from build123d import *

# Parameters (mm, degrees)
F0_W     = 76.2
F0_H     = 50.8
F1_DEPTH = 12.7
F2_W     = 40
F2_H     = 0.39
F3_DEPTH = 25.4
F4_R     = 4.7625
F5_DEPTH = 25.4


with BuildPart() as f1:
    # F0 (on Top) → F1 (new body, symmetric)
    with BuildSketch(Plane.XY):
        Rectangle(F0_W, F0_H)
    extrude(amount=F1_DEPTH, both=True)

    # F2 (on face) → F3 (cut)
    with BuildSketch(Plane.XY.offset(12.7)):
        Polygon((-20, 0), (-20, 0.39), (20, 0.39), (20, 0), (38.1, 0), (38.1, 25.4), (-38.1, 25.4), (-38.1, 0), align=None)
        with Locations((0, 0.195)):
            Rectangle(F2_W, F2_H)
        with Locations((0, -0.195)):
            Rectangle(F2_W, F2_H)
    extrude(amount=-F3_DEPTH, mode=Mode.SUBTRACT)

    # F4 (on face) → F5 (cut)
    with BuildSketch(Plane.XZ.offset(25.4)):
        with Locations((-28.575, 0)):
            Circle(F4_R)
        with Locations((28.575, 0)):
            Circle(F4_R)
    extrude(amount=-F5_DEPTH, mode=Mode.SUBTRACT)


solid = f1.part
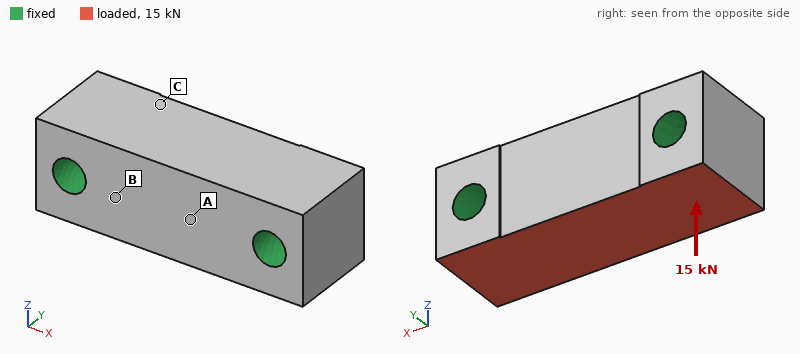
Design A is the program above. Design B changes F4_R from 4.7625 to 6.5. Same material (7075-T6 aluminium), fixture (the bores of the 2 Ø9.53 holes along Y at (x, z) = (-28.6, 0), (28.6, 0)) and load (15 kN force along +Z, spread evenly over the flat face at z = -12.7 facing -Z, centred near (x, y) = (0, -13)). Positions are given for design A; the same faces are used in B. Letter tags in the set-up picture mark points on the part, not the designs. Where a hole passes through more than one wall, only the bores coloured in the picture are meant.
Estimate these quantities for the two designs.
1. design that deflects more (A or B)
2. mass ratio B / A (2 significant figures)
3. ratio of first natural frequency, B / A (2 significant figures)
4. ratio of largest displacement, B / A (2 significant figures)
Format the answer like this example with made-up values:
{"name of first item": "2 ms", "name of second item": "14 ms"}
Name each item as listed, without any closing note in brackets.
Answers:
{"design that deflects more": "A", "mass ratio B / A": "0.93", "ratio of first natural frequency, B / A": "1.2", "ratio of largest displacement, B / A": "0.80"}
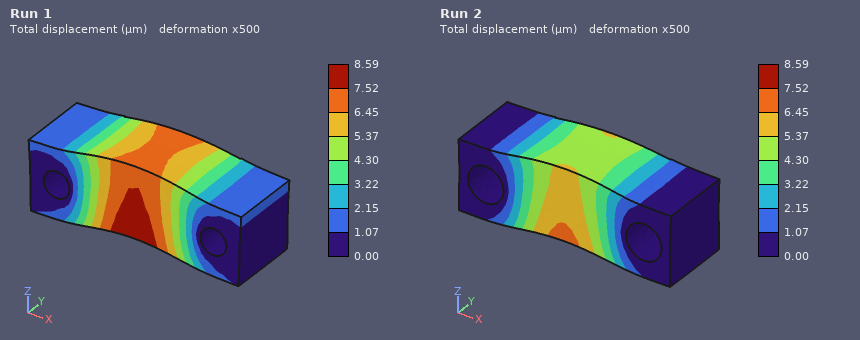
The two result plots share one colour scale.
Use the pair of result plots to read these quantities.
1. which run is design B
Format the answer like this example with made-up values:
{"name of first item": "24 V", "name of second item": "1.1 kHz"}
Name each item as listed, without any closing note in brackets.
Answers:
{"which run is design B": "Run 2"}
